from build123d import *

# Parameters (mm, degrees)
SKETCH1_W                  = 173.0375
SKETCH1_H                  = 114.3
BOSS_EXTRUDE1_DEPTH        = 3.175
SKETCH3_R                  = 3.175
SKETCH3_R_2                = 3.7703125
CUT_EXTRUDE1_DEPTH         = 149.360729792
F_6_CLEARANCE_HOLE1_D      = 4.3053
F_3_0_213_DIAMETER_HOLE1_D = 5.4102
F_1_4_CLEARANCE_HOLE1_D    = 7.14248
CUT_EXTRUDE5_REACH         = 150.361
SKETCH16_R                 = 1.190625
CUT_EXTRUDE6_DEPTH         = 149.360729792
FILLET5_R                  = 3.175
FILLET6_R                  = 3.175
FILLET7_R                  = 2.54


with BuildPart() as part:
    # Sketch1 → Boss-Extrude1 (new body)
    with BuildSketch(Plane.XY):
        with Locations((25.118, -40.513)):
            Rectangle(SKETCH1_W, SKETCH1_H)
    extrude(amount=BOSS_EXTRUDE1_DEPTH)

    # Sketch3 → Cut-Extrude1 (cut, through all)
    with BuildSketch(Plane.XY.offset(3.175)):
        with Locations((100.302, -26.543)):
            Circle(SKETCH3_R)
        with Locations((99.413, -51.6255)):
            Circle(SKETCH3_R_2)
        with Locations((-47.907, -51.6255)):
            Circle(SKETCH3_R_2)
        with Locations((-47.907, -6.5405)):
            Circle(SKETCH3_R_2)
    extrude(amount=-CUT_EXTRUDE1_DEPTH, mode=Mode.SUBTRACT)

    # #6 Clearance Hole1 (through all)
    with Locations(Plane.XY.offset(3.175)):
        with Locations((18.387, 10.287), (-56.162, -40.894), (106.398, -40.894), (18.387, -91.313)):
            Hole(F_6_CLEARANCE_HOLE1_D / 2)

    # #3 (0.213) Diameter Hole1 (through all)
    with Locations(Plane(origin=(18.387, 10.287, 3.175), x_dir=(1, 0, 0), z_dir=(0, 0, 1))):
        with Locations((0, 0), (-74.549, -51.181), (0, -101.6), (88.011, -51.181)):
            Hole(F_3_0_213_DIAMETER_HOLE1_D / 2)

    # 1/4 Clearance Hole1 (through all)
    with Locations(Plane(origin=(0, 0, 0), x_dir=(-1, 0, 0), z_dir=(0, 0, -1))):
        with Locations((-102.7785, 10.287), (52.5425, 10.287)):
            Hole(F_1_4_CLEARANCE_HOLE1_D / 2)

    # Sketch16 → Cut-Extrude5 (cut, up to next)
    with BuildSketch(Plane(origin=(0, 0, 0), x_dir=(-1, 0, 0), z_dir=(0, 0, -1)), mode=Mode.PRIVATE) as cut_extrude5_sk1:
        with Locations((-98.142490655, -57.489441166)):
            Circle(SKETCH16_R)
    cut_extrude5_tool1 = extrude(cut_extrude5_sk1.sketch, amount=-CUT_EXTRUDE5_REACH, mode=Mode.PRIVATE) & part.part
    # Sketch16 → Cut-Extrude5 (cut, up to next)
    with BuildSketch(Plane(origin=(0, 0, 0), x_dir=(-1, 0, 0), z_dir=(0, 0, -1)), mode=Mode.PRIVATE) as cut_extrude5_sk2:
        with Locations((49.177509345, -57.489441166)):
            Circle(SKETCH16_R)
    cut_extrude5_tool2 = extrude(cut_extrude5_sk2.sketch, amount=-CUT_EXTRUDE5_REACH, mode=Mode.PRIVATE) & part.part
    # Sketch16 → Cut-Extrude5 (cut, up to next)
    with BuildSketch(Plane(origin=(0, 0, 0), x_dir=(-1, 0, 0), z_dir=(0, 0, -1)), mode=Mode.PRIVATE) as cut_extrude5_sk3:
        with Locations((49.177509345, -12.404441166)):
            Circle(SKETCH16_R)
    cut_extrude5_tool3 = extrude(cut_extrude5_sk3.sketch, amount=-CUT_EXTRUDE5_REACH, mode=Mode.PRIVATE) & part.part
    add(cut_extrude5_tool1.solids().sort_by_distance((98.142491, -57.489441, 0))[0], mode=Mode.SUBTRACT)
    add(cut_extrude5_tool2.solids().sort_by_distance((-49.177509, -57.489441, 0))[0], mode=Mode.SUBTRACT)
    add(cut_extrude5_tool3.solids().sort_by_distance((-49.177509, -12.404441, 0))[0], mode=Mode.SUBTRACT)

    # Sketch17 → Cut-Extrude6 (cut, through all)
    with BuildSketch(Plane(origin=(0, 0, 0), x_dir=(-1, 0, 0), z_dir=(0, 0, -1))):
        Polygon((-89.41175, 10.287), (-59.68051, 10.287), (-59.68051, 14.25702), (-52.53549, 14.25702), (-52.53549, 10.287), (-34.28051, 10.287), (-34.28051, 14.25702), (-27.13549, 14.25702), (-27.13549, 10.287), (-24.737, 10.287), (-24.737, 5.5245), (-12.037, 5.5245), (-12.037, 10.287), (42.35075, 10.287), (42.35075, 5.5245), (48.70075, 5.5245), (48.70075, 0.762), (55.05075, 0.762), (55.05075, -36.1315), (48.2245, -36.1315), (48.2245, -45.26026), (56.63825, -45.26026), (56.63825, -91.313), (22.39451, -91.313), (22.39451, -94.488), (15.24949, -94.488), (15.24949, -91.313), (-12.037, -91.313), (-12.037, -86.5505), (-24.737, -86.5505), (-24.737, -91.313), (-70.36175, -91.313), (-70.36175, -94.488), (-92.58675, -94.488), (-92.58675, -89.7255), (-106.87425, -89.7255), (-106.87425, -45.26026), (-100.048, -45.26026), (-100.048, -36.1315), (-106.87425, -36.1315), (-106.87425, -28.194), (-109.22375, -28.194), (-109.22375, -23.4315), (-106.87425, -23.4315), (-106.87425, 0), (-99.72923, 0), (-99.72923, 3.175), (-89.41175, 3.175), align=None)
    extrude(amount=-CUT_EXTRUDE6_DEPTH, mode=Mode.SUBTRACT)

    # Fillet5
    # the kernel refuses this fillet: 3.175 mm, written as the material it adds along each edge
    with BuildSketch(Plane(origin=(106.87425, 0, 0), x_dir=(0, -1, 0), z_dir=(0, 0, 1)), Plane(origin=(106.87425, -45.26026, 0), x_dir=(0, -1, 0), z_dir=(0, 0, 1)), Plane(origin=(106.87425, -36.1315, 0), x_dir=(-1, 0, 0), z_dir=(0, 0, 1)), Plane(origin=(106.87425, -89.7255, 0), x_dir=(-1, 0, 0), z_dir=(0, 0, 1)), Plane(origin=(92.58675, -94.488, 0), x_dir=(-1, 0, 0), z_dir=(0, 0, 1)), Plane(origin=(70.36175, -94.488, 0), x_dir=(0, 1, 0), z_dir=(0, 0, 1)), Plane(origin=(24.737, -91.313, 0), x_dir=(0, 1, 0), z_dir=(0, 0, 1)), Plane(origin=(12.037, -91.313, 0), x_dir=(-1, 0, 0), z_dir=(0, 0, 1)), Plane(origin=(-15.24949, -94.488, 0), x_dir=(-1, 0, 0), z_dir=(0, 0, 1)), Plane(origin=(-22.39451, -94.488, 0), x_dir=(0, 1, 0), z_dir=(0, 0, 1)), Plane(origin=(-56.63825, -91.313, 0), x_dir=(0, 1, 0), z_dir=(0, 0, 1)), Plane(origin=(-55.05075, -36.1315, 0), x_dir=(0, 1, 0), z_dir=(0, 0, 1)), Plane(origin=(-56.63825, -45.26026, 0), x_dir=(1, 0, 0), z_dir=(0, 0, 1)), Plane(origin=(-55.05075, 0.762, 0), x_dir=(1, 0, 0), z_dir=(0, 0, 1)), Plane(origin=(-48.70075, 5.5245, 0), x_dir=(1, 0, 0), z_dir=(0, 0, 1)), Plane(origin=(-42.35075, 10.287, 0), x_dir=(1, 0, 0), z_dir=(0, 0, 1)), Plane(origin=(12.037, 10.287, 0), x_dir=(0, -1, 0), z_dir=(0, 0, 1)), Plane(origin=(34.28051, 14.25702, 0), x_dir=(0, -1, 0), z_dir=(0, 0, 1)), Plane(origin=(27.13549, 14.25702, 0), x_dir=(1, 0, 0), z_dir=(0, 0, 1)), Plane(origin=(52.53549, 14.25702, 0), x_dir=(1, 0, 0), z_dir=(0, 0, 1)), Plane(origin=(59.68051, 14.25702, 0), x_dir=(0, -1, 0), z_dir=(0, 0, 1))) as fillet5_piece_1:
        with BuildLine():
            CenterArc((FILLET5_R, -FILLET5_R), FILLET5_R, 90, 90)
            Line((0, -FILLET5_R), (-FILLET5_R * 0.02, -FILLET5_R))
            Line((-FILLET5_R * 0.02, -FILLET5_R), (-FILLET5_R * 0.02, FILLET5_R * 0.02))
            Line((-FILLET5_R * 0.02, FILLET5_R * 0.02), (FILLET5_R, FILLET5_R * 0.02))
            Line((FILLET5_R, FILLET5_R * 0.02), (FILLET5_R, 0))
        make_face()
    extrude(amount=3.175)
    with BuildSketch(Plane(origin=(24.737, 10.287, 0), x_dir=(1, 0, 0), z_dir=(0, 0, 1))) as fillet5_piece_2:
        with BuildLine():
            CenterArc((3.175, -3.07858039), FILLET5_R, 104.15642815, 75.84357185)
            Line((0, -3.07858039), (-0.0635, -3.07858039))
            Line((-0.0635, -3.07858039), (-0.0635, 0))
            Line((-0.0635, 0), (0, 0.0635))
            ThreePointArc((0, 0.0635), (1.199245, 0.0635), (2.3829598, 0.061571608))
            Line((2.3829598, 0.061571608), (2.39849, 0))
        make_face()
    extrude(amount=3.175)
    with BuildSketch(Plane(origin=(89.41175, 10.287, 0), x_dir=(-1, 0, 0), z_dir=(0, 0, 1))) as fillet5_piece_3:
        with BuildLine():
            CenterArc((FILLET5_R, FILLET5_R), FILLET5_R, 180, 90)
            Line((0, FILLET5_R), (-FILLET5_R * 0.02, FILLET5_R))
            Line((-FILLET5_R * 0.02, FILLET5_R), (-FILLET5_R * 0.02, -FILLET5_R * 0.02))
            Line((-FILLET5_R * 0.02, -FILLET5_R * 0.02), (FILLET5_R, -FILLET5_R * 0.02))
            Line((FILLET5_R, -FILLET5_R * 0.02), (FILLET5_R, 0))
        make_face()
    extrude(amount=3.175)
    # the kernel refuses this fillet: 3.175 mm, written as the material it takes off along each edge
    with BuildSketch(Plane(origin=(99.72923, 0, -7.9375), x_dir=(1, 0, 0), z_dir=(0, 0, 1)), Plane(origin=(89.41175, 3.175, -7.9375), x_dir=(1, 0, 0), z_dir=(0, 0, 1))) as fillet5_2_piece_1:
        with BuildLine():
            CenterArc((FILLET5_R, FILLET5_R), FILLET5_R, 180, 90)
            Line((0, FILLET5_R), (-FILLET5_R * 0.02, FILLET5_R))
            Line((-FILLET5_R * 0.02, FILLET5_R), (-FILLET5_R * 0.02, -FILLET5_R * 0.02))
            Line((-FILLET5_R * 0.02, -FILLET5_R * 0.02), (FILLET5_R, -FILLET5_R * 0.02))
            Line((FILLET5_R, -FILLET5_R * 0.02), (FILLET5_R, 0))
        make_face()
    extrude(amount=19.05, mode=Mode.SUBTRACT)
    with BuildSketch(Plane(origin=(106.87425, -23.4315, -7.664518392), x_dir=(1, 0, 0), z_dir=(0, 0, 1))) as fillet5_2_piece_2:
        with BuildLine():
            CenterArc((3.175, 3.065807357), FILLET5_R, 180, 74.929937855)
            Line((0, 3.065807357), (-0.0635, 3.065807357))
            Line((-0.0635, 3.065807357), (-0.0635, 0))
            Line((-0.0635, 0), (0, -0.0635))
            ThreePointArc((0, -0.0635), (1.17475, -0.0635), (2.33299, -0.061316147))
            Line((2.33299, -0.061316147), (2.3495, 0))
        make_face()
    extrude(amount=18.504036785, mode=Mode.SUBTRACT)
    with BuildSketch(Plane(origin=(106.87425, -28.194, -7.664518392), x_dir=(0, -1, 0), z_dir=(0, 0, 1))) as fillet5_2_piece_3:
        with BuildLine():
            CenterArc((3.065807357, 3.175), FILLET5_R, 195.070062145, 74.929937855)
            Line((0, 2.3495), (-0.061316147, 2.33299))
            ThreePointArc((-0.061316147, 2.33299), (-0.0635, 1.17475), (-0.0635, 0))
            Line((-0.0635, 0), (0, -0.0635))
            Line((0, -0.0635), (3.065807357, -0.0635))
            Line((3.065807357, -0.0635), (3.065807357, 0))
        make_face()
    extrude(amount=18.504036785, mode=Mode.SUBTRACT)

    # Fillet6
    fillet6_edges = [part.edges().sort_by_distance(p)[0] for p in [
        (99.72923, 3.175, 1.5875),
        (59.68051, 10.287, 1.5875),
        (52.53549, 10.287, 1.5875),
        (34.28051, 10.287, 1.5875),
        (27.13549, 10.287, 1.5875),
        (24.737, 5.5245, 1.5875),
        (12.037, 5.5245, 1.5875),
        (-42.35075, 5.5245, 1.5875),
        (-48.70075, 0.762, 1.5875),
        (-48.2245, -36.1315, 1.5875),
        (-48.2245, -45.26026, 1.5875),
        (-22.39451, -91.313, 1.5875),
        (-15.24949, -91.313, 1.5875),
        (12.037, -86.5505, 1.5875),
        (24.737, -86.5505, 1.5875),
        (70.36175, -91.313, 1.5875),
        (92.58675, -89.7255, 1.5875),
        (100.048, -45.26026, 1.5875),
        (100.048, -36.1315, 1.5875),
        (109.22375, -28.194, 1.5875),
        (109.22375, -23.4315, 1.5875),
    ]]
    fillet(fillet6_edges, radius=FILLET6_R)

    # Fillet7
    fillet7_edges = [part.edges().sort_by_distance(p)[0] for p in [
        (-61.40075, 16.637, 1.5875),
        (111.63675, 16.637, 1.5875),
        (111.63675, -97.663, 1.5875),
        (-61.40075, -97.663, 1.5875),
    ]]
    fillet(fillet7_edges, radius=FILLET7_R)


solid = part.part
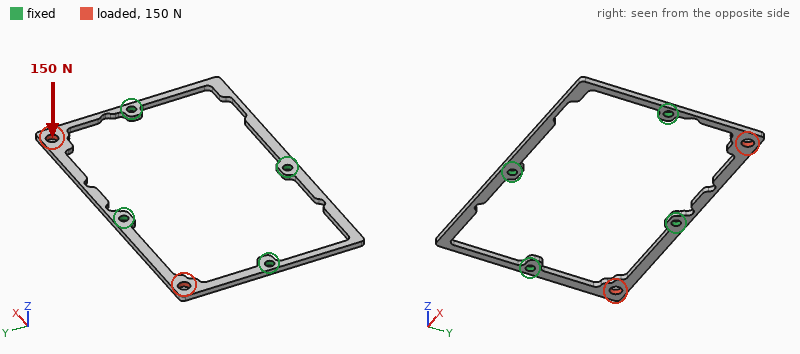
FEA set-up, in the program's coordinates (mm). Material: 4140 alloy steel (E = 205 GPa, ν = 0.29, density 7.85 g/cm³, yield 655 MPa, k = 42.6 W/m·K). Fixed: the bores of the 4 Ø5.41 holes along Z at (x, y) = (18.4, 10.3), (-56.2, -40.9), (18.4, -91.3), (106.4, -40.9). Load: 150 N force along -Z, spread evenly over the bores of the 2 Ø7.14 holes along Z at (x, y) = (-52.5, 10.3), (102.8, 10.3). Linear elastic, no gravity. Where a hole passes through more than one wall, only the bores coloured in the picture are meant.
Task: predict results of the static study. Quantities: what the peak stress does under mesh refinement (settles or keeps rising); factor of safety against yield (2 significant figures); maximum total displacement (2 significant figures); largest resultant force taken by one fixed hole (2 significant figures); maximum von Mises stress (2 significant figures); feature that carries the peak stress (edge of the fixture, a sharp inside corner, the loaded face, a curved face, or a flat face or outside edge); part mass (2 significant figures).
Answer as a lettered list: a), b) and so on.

a) settles
b) 1.5
c) 0.77 mm
d) 54 N
e) 440 MPa
f) a curved face
g) 86 g
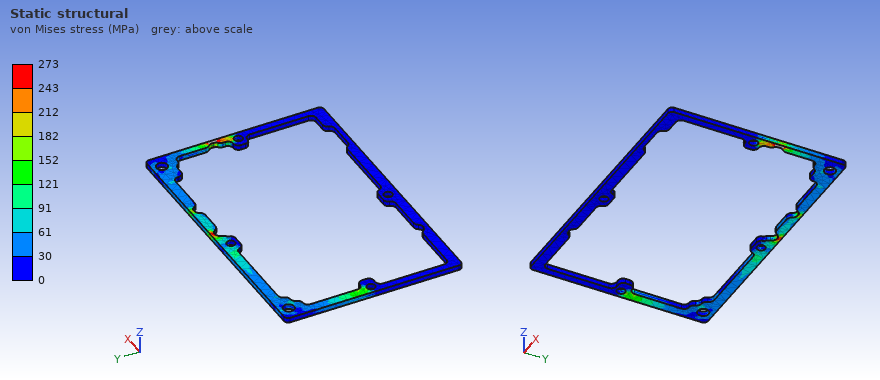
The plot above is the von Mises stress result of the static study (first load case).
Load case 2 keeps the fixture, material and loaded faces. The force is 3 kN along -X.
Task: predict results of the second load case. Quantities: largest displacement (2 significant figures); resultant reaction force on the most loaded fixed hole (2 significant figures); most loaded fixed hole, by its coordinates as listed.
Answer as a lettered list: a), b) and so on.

a) 0.12 mm
b) 2.8 kN
c) (18.4, 10.3)
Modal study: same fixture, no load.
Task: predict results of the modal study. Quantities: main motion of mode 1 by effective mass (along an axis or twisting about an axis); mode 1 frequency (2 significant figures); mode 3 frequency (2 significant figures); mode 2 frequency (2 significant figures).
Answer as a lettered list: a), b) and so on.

a) along Z
b) 570 Hz
c) 830 Hz
d) 710 Hz
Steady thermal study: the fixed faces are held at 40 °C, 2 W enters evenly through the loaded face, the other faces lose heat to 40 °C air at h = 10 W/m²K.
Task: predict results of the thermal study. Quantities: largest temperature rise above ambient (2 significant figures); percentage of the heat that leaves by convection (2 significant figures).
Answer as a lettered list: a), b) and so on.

a) 30 K
b) 39 %
